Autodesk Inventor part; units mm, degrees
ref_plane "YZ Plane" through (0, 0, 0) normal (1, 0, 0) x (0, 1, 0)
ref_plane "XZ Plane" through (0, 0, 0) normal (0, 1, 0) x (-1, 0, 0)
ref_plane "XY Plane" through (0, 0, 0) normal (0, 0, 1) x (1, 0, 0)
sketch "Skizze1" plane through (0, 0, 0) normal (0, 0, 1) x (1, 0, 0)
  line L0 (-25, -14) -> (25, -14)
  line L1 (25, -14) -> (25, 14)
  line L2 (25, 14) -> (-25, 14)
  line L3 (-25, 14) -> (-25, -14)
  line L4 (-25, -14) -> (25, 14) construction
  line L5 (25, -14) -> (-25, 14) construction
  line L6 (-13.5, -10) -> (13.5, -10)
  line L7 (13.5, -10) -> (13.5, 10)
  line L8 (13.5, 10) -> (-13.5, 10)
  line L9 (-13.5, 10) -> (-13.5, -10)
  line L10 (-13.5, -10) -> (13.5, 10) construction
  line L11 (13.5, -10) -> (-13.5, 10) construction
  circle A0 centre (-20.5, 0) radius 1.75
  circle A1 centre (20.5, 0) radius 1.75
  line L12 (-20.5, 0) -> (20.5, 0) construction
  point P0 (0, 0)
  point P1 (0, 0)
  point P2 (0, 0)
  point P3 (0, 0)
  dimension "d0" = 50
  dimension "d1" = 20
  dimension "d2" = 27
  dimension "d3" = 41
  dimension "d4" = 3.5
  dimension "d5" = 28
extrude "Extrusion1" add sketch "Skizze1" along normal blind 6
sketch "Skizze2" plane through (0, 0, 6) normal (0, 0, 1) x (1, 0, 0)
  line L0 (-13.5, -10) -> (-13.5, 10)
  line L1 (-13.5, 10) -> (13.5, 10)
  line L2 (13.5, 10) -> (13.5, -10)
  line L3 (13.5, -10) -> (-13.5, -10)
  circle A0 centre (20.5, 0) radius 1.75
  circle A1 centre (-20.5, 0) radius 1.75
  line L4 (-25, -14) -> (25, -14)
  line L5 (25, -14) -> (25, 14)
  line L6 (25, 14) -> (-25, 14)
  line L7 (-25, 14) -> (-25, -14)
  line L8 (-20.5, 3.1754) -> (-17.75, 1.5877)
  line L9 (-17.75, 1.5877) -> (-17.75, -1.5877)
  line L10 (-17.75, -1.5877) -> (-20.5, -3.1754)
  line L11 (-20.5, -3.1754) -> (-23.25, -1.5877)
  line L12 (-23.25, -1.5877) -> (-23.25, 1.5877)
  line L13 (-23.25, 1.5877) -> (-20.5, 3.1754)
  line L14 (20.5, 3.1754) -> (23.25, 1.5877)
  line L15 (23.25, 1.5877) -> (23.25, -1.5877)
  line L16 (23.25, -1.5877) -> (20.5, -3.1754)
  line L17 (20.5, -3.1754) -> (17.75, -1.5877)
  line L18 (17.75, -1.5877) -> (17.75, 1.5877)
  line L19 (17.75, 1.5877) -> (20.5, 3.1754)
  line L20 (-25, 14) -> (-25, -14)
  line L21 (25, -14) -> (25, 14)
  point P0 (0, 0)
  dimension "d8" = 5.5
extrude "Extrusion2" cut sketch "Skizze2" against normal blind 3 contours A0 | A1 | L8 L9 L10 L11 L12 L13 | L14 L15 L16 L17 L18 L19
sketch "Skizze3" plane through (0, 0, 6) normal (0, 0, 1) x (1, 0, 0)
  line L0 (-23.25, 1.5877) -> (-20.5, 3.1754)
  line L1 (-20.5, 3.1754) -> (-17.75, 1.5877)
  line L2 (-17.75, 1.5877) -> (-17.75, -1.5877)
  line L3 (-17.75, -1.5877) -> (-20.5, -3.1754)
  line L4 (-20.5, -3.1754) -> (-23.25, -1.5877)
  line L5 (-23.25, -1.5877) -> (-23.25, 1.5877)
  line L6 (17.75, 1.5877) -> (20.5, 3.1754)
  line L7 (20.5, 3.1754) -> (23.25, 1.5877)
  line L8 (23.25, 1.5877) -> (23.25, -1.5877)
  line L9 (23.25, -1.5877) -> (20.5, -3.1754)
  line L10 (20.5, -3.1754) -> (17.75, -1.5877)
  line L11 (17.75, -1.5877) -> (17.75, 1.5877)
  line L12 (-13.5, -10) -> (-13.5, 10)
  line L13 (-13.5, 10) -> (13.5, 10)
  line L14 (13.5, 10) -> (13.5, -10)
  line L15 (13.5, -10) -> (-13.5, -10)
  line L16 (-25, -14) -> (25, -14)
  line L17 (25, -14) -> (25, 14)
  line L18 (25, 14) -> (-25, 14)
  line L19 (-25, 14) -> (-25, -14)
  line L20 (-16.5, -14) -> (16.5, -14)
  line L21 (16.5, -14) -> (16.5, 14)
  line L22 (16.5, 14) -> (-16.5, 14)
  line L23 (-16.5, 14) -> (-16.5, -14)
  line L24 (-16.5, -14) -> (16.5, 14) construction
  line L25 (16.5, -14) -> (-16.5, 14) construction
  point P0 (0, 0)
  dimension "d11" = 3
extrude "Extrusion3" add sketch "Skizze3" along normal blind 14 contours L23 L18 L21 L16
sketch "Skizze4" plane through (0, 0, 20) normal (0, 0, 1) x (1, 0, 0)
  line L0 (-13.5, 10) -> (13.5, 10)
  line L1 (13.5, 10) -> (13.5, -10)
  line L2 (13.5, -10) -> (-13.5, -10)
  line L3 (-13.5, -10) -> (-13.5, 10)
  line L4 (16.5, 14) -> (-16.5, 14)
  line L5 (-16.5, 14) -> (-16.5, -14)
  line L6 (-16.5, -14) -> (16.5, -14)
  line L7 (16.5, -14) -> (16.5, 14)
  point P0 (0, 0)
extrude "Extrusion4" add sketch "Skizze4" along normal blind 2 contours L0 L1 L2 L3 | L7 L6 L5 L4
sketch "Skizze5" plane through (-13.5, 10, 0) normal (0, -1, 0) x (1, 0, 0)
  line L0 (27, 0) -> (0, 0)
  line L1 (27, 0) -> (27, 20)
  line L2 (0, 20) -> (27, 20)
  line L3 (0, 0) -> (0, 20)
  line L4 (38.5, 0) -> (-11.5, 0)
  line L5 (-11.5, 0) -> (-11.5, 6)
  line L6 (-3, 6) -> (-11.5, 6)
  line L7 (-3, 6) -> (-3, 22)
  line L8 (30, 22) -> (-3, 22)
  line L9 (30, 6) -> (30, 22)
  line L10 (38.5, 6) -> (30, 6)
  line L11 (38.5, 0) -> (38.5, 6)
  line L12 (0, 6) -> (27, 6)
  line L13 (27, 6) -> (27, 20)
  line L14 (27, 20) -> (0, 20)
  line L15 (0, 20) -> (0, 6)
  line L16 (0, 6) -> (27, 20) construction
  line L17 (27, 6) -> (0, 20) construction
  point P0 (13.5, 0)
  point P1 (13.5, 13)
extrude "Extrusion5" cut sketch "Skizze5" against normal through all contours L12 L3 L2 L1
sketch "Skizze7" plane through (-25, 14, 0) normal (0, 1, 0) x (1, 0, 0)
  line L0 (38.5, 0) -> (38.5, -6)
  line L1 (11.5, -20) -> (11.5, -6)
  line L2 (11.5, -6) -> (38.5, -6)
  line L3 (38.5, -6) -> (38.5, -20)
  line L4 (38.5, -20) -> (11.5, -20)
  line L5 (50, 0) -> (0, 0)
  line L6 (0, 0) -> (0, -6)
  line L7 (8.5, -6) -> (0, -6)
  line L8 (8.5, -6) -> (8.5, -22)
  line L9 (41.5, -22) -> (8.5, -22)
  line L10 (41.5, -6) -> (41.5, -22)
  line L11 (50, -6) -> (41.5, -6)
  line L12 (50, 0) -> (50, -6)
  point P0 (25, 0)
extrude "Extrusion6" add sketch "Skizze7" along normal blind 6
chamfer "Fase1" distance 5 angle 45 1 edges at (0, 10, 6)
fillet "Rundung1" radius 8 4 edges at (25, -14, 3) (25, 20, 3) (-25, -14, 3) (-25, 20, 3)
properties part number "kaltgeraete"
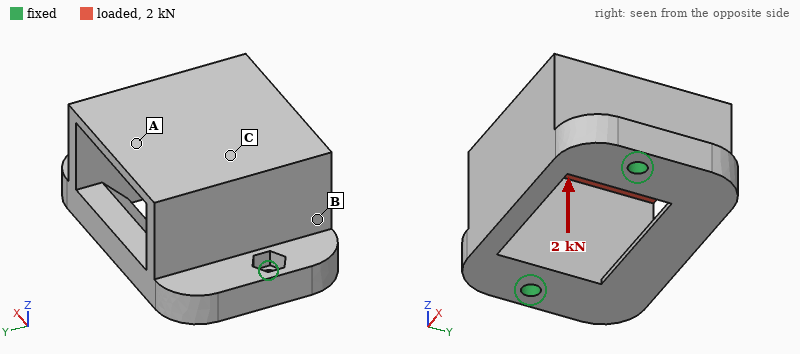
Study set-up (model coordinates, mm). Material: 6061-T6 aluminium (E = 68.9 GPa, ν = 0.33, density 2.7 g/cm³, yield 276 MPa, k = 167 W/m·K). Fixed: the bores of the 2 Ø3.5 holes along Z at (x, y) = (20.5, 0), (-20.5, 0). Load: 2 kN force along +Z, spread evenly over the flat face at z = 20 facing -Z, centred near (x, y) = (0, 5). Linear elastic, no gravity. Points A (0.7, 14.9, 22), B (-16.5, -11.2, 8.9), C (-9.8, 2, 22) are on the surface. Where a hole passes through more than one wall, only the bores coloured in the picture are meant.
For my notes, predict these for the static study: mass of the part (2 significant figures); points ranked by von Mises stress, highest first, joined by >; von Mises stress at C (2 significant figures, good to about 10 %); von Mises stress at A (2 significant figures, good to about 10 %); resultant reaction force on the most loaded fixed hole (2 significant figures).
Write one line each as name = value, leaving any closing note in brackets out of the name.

mass of the part = 34 g
points ranked by von Mises stress, highest first, joined by > = A > C > B
von Mises stress at C = 46 MPa
von Mises stress at A = 130 MPa
resultant reaction force on the most loaded fixed hole = 1.1 kN
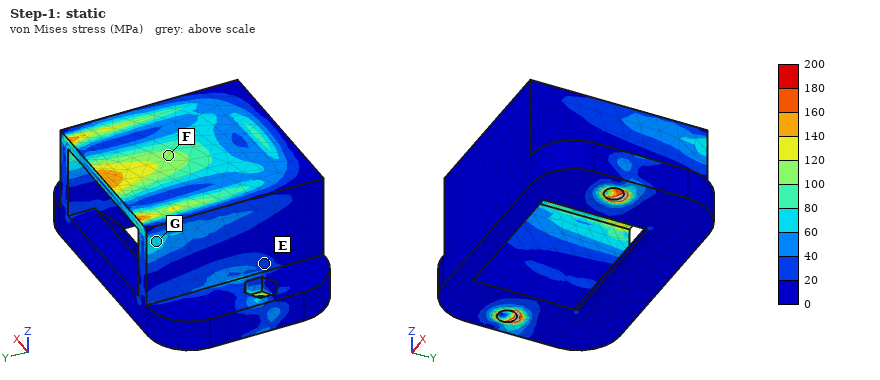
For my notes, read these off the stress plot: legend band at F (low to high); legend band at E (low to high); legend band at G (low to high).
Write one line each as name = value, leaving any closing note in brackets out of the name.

legend band at F = 100 to 120 MPa
legend band at E = 20 to 40 MPa
legend band at G = 60 to 80 MPa
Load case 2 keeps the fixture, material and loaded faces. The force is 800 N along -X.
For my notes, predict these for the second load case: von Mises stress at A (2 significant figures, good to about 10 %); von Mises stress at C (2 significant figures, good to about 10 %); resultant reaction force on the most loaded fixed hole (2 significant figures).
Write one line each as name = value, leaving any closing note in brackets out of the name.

von Mises stress at A = 12 MPa
von Mises stress at C = 21 MPa
resultant reaction force on the most loaded fixed hole = 540 N
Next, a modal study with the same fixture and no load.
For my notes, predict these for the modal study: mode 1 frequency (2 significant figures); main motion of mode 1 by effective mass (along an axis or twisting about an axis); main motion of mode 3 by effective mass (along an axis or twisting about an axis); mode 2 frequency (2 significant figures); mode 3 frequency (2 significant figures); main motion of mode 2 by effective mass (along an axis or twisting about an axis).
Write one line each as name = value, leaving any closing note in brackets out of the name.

mode 1 frequency = 3200 Hz
main motion of mode 1 by effective mass = along Y
main motion of mode 3 by effective mass = along Z
mode 2 frequency = 6800 Hz
mode 3 frequency = 11 kHz
main motion of mode 2 by effective mass = along X
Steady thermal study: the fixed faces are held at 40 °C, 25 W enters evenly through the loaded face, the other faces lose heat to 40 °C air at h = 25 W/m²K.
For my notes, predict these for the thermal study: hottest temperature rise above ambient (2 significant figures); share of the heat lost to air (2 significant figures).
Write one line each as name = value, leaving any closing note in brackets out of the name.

hottest temperature rise above ambient = 25 K
share of the heat lost to air = 7.7 %
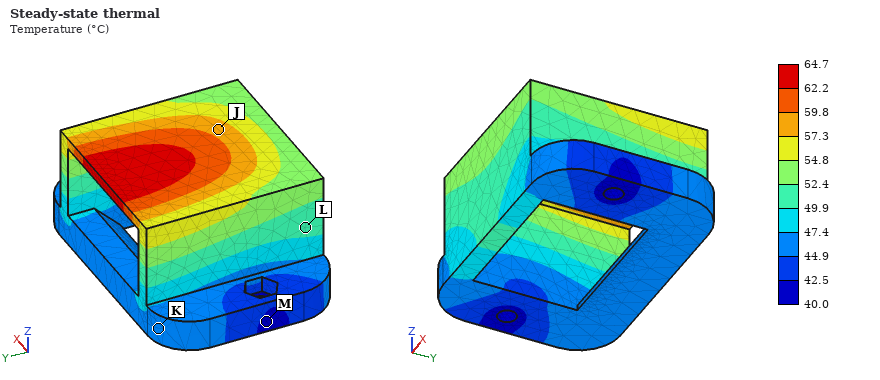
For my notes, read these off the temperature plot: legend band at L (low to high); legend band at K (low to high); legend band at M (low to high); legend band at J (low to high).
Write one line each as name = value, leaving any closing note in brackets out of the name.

legend band at L = 49.9 to 52.4 °C
legend band at K = 44.9 to 47.4 °C
legend band at M = 40.0 to 42.5 °C
legend band at J = 57.3 to 59.8 °C
